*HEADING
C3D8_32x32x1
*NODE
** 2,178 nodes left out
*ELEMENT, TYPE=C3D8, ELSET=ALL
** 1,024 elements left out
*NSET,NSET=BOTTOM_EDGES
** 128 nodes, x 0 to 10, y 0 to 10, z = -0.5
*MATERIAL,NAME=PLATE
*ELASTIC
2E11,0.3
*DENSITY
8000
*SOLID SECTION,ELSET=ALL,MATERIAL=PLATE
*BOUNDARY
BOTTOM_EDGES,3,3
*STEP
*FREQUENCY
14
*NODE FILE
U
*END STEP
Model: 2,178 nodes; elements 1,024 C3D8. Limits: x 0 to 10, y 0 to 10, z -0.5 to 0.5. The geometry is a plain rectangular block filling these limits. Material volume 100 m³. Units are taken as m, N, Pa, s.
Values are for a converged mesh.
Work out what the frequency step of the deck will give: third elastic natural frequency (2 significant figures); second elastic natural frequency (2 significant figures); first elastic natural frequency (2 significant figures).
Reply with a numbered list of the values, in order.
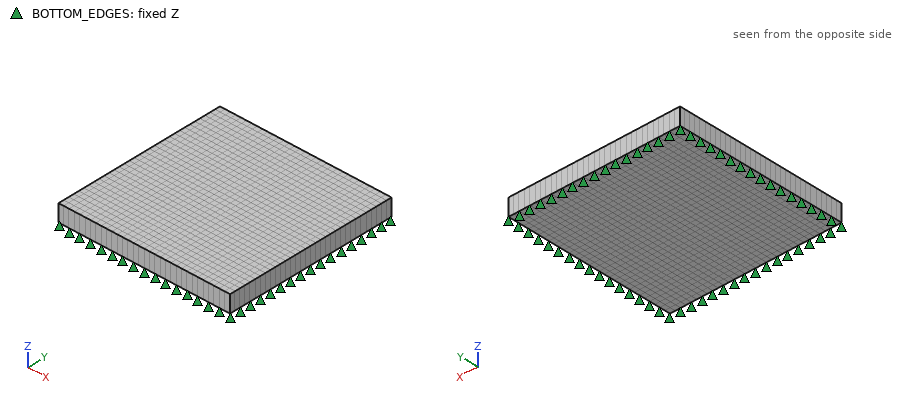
1. 100 Hz
2. 100 Hz
3. 43 Hz
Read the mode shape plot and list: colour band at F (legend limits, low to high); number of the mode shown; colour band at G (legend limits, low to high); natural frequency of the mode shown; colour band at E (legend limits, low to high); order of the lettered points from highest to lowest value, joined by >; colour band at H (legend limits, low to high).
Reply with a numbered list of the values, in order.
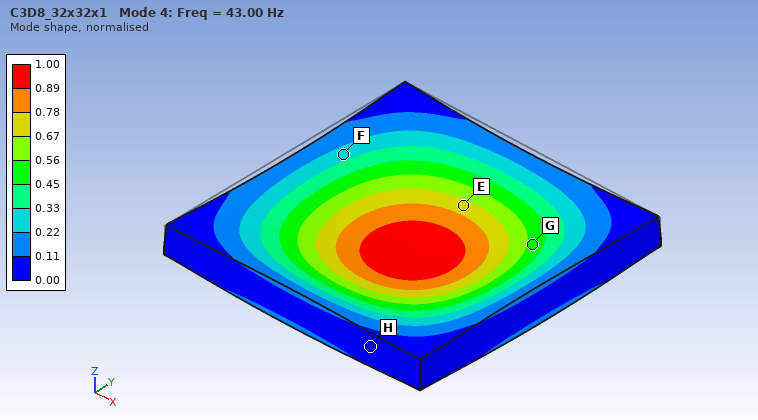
1. 0.22 to 0.33
2. 4
3. 0.45 to 0.56
4. 43.00 Hz
5. 0.67 to 0.78
6. E > G > F > H
7. 0.00 to 0.11
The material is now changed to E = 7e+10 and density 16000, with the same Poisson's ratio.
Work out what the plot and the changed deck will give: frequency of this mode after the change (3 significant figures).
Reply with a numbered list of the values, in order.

1. 18.0 Hz
